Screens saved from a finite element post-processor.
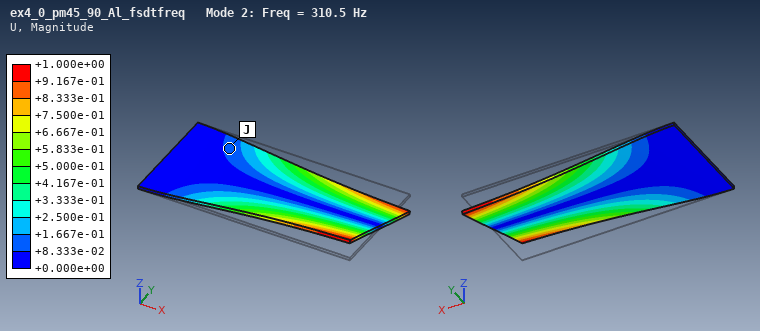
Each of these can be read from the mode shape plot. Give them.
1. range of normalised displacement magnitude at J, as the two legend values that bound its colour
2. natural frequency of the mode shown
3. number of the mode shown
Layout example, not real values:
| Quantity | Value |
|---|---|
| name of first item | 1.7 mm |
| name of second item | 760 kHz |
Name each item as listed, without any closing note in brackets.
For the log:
| Quantity | Value |
|---|---|
| range of normalised displacement magnitude at J, as the two legend values that bound its colour | +8.333e-02 to +1.667e-01 |
| natural frequency of the mode shown | 310.5 Hz |
| number of the mode shown | 2 |
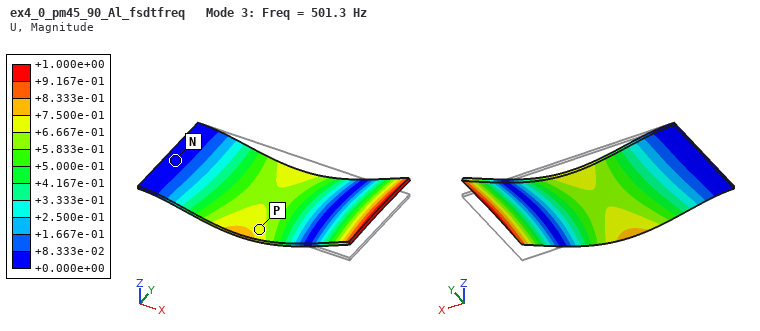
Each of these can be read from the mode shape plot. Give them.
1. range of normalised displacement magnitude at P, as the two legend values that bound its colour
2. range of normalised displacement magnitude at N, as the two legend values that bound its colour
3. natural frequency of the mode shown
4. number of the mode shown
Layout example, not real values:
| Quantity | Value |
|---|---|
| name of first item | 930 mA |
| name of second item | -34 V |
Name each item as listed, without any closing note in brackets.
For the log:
| Quantity | Value |
|---|---|
| range of normalised displacement magnitude at P, as the two legend values that bound its colour | +6.667e-01 to +7.500e-01 |
| range of normalised displacement magnitude at N, as the two legend values that bound its colour | +0.000e+00 to +8.333e-02 |
| natural frequency of the mode shown | 501.3 Hz |
| number of the mode shown | 3 |
